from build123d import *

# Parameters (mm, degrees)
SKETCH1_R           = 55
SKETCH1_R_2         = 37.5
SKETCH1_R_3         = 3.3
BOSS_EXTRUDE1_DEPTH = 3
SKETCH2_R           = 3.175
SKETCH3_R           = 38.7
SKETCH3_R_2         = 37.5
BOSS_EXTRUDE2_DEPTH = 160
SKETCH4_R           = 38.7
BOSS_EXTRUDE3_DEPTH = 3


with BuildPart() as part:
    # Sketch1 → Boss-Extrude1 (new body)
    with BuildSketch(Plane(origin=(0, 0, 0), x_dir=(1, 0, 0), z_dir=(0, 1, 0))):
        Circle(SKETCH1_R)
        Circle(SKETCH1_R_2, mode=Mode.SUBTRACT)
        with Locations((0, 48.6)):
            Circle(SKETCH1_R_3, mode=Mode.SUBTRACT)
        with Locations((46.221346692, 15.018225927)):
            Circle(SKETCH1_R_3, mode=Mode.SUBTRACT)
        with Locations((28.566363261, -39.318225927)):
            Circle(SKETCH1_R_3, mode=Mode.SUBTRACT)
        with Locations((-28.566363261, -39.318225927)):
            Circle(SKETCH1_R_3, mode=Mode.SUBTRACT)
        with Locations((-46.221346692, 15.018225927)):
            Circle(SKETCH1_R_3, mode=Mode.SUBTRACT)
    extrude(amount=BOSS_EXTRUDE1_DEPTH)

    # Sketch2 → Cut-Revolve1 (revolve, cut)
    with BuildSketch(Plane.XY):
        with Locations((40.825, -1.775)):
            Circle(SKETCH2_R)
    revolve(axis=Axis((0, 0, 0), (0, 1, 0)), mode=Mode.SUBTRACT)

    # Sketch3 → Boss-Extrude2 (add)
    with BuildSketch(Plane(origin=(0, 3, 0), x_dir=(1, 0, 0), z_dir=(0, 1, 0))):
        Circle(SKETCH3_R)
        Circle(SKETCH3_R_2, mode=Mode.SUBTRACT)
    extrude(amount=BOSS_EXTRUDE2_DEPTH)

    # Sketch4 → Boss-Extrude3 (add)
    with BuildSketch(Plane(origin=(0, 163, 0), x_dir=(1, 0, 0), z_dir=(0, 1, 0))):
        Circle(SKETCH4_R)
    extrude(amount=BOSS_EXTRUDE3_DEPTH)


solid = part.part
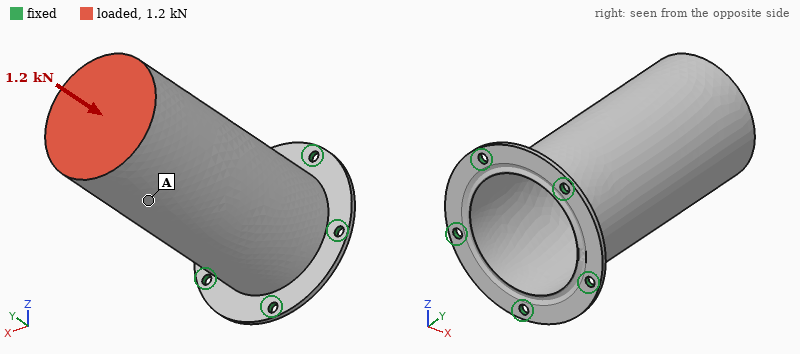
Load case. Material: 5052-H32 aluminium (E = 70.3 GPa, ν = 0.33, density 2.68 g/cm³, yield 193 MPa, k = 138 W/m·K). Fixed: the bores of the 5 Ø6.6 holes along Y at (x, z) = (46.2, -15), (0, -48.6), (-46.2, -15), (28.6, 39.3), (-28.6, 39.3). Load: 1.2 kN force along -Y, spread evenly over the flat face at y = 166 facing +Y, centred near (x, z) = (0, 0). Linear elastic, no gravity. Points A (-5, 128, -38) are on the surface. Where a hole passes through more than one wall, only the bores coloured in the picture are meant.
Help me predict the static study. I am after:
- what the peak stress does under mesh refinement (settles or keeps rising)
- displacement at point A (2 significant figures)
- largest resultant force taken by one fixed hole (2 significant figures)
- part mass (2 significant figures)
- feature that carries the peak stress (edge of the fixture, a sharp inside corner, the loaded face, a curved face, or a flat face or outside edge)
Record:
keeps rising
0.024 mm
260 N
200 g
edge of the fixture
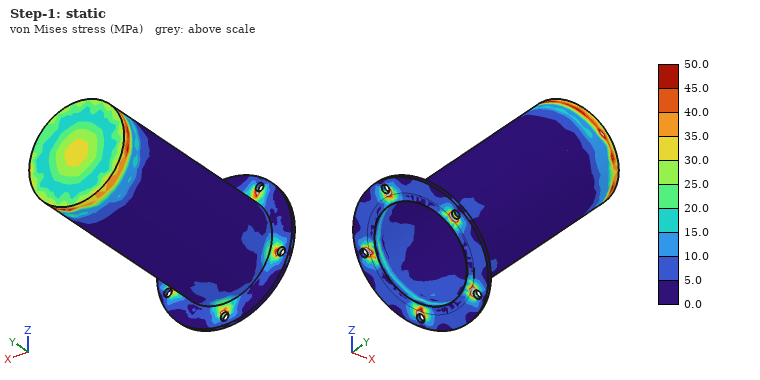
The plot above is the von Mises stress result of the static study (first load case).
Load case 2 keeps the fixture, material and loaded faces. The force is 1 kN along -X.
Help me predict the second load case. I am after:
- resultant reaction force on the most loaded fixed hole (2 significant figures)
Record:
1.6 kN
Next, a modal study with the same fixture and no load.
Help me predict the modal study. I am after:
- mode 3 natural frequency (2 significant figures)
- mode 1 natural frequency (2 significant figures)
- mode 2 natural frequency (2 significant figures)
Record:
2200 Hz
740 Hz
750 Hz
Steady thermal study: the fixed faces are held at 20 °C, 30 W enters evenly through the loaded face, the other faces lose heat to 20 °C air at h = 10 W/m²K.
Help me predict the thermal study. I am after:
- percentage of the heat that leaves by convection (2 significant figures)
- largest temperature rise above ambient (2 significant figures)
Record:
73 %
64 K
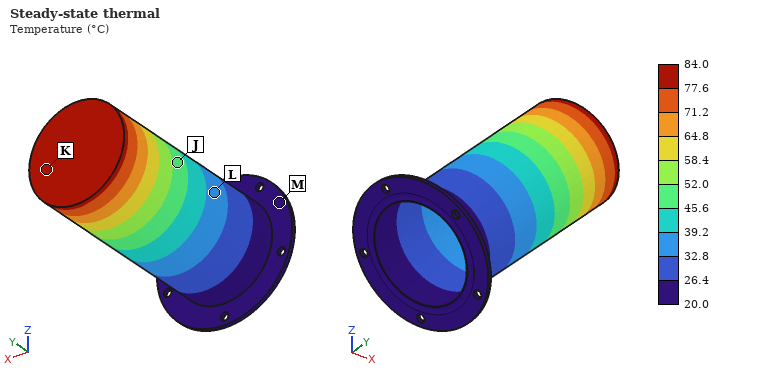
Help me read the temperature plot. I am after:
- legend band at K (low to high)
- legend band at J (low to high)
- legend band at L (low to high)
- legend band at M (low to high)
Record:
77.6 to 84.0 °C
45.6 to 52.0 °C
32.8 to 39.2 °C
20.0 to 26.4 °C
